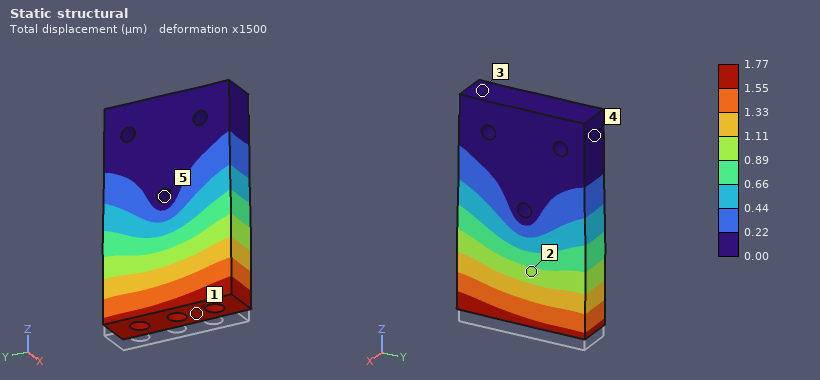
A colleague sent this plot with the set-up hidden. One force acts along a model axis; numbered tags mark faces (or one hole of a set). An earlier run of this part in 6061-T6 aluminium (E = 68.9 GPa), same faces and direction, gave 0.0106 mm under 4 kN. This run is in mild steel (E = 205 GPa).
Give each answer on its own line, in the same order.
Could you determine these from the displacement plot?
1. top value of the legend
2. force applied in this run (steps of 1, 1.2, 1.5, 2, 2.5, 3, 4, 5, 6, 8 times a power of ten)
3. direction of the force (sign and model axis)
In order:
1.77 µm
2 kN
+Z
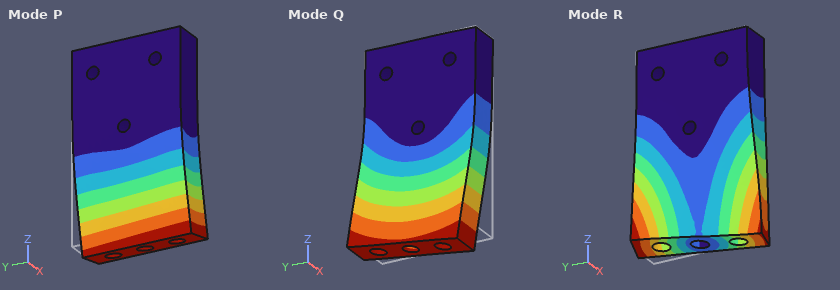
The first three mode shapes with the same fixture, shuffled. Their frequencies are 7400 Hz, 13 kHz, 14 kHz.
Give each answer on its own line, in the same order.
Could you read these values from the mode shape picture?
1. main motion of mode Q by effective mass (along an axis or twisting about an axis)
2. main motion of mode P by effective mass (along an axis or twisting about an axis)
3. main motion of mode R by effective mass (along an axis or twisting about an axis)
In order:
along Y
along X
twisting about Z
